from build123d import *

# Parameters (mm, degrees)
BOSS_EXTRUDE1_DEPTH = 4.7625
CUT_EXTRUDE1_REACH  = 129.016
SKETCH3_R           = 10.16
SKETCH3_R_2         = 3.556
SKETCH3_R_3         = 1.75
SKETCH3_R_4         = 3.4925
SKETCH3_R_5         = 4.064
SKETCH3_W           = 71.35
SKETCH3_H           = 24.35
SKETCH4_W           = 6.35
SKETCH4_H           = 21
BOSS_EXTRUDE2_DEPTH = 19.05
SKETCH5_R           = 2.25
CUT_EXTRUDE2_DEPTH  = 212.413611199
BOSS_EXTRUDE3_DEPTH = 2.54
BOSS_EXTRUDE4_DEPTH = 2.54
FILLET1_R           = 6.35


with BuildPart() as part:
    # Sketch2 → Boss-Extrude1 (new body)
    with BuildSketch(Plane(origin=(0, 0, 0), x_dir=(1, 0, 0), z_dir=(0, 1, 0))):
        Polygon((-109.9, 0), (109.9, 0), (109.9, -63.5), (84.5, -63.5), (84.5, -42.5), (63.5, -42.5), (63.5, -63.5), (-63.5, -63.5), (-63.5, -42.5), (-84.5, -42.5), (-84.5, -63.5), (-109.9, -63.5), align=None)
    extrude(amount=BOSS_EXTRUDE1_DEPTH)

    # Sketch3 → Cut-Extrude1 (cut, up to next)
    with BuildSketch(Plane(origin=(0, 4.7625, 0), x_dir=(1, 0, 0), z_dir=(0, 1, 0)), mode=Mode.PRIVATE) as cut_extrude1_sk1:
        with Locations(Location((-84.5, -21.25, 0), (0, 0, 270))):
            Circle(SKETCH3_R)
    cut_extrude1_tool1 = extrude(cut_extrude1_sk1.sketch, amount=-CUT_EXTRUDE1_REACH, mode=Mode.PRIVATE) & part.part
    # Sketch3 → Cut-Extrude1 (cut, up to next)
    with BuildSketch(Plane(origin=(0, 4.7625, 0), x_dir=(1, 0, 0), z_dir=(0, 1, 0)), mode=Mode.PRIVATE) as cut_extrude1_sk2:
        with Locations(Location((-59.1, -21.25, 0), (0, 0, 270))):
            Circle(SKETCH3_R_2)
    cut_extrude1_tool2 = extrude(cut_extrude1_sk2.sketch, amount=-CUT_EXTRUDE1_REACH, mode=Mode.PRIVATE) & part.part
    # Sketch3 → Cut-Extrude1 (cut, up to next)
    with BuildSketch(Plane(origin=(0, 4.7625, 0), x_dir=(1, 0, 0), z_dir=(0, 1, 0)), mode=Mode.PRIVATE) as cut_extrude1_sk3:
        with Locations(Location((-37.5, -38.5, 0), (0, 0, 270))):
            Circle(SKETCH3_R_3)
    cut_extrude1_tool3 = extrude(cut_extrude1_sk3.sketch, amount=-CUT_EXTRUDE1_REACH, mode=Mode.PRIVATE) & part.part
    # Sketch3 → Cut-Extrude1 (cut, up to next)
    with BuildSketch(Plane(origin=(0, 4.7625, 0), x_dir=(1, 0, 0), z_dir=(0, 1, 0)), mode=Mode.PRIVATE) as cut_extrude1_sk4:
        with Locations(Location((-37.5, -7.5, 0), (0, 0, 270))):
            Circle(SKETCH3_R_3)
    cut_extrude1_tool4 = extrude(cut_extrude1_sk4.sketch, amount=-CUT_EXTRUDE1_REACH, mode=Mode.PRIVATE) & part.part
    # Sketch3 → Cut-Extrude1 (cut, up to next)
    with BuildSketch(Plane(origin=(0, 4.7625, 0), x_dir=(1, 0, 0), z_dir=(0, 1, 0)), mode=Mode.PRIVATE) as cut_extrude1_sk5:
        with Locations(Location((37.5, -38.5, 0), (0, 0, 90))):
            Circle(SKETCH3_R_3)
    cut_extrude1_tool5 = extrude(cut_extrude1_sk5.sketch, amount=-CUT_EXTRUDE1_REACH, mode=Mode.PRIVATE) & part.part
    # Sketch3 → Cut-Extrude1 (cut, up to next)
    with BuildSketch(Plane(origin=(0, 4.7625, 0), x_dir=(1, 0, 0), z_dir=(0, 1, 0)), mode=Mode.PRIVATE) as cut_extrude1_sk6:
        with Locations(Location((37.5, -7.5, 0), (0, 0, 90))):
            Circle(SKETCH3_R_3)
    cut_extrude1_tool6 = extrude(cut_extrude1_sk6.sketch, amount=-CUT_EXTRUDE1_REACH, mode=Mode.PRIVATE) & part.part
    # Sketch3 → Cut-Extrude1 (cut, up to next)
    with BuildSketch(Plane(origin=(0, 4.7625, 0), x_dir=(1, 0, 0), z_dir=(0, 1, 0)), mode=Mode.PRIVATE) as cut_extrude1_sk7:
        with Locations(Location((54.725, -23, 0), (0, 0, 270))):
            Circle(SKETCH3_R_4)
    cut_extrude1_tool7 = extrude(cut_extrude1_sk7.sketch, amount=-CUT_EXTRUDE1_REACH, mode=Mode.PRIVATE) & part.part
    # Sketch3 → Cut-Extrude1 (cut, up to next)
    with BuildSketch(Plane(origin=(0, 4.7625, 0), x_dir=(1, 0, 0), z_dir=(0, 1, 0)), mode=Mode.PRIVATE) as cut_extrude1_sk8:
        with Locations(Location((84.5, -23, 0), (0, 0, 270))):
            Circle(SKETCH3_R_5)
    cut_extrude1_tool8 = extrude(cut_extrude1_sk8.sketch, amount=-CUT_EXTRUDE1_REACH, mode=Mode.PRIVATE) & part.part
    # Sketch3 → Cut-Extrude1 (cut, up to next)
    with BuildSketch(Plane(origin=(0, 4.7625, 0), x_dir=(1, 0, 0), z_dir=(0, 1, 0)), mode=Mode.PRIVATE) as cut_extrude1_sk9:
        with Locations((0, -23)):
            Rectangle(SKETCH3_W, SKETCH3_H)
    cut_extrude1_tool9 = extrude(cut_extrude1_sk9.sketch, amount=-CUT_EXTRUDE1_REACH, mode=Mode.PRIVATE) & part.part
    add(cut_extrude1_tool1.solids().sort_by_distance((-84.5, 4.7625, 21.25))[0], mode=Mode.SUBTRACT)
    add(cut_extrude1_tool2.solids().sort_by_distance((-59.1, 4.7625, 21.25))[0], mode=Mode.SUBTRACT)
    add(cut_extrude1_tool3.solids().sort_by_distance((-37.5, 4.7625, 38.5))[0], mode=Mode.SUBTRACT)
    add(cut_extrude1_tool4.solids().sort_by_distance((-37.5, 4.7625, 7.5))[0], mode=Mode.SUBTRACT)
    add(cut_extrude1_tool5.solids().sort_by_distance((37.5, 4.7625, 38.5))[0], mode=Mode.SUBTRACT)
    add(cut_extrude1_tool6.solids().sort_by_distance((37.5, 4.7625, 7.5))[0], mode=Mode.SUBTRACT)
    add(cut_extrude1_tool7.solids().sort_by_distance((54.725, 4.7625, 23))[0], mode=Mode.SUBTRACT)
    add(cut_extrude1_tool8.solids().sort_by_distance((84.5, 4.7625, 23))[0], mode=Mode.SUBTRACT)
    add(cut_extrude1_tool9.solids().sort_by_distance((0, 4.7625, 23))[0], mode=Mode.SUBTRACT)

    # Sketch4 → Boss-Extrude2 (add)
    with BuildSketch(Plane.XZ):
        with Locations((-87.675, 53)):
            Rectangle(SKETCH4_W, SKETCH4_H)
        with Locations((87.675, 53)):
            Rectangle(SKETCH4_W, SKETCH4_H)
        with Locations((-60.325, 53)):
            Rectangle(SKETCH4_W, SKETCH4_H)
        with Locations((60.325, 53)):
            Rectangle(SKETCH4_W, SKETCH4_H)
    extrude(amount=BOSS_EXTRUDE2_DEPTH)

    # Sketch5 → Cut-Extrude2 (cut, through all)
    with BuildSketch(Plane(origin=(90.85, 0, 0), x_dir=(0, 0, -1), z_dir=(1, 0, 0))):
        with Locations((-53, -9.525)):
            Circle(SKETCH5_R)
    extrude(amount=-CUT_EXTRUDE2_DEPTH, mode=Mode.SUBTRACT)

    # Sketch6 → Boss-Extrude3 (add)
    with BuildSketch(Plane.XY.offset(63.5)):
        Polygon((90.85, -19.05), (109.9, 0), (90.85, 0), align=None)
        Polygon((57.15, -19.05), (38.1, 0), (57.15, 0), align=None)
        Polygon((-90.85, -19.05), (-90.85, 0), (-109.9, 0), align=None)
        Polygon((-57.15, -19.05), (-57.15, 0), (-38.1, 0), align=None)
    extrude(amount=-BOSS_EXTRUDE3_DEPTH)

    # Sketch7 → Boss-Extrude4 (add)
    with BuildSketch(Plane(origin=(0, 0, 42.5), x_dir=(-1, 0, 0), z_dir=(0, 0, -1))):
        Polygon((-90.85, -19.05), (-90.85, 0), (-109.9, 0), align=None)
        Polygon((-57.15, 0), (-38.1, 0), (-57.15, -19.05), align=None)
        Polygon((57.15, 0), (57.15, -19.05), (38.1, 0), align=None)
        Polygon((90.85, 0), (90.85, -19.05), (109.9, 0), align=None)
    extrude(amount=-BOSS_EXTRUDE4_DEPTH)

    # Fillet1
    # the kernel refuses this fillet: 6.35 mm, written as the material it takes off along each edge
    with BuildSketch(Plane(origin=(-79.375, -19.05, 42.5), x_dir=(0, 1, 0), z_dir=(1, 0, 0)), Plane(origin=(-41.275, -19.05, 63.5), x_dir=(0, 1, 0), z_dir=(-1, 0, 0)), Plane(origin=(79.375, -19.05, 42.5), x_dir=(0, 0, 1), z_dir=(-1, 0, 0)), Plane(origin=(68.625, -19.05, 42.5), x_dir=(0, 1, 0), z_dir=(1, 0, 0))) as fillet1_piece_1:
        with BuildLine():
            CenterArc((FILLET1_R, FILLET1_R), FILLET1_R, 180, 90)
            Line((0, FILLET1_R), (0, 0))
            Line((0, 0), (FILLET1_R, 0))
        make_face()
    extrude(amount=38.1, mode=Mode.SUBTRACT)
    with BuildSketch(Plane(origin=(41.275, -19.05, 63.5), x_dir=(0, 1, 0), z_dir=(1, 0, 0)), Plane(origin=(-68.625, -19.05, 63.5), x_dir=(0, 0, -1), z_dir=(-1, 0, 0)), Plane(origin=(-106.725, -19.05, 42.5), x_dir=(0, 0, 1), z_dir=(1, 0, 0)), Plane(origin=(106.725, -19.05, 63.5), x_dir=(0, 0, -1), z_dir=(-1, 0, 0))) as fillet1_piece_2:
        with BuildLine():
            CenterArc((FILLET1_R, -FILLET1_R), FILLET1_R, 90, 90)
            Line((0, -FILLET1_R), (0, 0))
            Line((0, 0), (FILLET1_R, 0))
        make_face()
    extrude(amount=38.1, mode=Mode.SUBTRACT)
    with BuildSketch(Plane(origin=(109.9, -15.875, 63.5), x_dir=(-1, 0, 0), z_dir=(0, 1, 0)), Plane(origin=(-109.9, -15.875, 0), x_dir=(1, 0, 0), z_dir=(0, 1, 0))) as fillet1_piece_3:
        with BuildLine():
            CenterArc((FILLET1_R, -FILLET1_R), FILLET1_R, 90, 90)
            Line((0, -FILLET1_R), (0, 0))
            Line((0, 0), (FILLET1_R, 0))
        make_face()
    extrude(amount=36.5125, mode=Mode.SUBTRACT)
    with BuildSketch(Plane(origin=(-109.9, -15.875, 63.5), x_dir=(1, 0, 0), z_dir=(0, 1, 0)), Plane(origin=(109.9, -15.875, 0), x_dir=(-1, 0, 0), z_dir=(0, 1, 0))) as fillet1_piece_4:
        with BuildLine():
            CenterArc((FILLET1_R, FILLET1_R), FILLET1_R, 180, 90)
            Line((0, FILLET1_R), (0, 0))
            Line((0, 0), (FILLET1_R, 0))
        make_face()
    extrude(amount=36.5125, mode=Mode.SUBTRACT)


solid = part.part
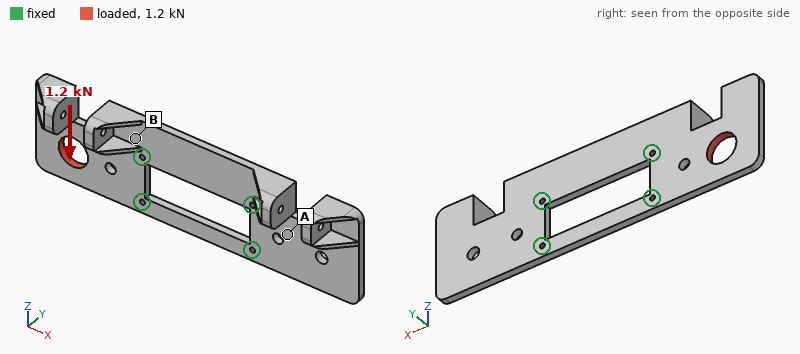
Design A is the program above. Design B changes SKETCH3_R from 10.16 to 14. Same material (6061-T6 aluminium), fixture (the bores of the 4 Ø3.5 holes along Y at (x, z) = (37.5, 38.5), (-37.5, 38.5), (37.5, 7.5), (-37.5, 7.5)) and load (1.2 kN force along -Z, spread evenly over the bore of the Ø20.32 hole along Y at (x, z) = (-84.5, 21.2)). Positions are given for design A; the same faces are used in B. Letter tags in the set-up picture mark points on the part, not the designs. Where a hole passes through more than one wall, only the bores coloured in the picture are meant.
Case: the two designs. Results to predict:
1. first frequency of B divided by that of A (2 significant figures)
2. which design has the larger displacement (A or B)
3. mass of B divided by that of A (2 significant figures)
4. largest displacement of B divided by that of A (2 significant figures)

0.98
B
0.98
1.5
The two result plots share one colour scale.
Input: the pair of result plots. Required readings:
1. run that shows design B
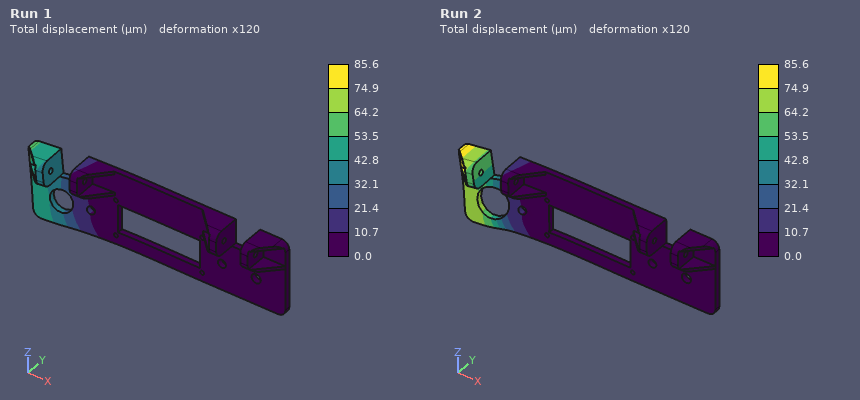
Run 2
